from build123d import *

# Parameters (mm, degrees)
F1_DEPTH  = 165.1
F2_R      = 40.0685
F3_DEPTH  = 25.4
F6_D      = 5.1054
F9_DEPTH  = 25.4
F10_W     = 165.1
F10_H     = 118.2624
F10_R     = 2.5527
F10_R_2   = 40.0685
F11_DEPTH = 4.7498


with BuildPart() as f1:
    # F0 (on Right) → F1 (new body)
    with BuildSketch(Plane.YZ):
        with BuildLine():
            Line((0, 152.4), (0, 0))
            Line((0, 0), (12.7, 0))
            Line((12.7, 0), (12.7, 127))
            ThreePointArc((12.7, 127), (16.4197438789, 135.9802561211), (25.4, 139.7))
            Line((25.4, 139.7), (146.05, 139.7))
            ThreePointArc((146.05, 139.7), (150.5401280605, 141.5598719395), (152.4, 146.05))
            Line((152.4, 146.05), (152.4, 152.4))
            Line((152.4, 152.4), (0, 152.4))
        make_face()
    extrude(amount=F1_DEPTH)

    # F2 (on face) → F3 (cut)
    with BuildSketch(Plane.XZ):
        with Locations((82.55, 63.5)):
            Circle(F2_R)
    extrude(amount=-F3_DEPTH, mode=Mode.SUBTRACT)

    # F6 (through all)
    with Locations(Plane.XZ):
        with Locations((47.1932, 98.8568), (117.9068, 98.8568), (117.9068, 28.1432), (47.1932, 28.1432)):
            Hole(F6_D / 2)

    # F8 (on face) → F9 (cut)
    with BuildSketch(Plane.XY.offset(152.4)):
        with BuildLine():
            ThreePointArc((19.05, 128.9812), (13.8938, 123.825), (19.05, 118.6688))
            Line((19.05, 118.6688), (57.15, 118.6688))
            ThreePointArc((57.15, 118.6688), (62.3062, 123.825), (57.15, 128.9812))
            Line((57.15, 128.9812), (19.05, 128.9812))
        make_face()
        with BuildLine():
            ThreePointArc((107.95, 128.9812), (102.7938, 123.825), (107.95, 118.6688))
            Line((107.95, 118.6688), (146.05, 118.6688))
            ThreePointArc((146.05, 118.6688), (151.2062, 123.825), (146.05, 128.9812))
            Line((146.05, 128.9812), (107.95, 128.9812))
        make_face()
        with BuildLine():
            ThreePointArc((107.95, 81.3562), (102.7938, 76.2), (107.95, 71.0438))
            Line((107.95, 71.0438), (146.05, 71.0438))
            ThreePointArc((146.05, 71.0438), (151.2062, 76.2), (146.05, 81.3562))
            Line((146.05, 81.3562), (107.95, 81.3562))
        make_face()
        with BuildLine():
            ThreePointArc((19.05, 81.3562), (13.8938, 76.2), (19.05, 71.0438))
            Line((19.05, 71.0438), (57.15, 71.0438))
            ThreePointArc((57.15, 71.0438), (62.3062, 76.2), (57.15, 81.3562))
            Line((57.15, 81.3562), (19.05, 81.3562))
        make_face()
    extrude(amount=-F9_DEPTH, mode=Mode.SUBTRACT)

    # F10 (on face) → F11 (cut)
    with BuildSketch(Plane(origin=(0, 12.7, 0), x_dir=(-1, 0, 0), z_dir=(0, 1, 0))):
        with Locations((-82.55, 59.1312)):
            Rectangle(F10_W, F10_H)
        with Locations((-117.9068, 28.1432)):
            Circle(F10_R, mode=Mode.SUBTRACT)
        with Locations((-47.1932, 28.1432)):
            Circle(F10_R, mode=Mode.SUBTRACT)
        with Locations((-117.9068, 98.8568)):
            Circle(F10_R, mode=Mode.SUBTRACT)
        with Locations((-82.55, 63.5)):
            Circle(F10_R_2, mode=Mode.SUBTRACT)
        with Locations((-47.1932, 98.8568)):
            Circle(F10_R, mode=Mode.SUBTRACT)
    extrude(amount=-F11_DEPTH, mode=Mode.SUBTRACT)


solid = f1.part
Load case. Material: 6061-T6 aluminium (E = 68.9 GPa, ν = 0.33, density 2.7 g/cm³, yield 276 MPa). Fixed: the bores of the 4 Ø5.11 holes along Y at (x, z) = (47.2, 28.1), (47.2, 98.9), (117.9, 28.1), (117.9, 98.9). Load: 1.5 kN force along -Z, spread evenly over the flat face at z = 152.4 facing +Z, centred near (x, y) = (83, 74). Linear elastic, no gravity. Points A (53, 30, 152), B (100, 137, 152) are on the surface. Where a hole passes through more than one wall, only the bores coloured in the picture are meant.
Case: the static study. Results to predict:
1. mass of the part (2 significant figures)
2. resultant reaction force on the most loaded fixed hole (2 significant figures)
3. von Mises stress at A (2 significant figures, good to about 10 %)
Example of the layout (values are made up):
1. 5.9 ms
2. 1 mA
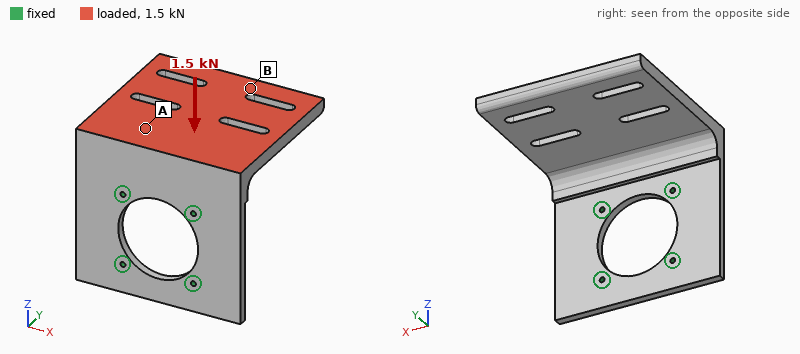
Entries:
1. 1.2 kg
2. 740 N
3. 14 MPa
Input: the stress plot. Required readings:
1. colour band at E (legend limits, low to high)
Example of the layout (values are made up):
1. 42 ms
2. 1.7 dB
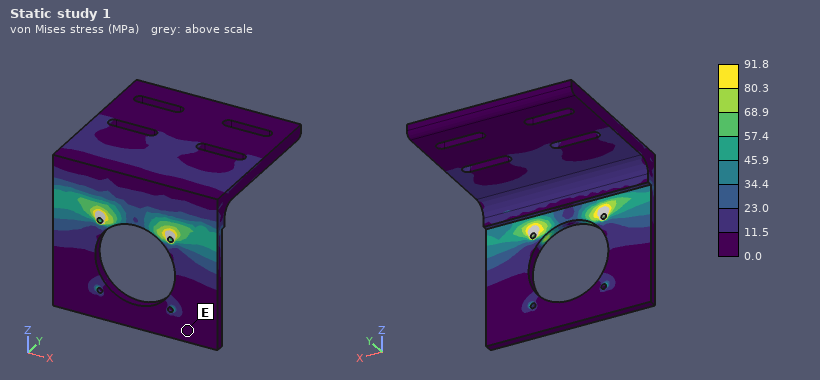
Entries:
1. 0.0 to 11.5 MPa
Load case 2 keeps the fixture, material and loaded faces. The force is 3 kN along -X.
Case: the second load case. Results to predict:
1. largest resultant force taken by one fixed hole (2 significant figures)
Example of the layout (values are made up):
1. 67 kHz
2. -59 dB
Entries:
1. 3.5 kN
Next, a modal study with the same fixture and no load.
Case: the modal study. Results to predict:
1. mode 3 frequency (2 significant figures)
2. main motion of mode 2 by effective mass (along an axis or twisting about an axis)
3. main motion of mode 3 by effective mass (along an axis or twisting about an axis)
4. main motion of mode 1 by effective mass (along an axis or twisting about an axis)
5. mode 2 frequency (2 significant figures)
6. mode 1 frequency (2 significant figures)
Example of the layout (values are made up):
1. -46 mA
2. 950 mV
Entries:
1. 1000 Hz
2. along X
3. along Y
4. along Z
5. 520 Hz
6. 210 Hz
